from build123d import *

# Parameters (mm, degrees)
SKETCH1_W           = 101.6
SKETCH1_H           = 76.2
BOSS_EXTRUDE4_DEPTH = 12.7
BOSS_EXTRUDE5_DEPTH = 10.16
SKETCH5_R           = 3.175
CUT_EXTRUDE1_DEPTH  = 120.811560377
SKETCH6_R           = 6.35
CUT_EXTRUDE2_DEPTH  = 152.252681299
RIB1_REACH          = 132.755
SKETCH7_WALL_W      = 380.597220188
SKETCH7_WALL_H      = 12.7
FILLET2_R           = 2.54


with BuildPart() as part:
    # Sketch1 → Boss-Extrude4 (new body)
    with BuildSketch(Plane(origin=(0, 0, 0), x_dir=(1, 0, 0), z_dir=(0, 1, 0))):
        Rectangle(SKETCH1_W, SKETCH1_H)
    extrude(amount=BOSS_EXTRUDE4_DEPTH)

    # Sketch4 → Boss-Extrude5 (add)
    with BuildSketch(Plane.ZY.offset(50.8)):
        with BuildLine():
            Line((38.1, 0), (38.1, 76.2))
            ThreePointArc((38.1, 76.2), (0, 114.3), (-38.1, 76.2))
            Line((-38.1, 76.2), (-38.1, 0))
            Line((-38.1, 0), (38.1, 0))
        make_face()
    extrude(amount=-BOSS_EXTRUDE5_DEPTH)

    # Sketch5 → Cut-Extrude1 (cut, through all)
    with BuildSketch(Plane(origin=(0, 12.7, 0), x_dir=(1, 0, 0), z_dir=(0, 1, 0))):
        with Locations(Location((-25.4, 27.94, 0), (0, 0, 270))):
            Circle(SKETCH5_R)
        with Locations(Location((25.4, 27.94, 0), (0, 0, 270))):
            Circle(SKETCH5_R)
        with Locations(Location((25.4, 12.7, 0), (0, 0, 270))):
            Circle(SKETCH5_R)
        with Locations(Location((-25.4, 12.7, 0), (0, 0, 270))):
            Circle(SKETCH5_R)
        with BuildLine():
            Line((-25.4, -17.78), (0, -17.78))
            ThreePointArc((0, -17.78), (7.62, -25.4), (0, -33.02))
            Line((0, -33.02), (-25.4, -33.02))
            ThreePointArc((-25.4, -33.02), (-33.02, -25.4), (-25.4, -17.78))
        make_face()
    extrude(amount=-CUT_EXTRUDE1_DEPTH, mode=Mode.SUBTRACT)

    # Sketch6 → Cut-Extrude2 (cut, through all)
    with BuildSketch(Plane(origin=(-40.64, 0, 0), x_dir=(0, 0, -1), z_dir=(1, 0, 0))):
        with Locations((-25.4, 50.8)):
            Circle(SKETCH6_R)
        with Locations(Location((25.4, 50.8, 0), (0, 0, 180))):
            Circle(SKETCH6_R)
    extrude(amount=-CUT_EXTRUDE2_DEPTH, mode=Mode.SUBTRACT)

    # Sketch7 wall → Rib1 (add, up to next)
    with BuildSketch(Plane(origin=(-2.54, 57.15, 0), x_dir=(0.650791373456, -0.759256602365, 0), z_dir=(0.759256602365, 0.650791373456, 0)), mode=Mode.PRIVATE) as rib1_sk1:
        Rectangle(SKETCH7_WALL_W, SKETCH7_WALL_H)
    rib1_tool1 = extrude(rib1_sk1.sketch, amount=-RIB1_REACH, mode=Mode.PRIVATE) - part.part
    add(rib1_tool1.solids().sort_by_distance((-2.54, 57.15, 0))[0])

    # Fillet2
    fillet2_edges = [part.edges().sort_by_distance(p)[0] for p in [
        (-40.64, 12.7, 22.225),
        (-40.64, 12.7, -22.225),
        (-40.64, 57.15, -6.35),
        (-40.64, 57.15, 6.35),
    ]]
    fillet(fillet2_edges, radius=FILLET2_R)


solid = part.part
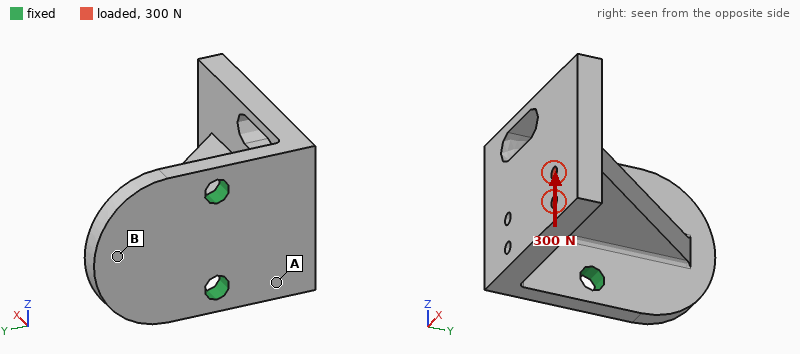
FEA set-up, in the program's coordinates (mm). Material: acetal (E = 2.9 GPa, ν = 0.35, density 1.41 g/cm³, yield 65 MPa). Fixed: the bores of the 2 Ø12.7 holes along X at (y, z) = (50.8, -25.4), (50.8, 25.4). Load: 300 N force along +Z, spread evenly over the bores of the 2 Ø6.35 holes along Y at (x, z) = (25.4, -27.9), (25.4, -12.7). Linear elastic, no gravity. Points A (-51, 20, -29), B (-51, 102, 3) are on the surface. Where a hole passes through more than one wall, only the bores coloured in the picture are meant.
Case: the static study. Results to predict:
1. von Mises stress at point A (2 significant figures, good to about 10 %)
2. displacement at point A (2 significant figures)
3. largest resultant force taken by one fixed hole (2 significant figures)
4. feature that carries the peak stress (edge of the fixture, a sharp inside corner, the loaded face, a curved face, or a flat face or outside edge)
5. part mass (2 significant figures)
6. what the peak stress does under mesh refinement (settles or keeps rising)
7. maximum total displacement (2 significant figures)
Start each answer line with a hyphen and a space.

- 4.1 MPa
- 0.15 mm
- 540 N
- edge of the fixture
- 290 g
- keeps rising
- 0.76 mm
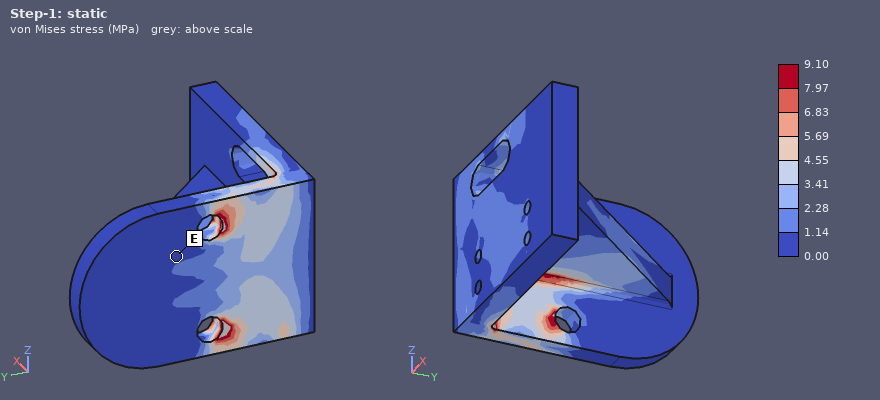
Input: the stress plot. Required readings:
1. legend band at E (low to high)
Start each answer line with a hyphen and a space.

- 0.00 to 1.14 MPa
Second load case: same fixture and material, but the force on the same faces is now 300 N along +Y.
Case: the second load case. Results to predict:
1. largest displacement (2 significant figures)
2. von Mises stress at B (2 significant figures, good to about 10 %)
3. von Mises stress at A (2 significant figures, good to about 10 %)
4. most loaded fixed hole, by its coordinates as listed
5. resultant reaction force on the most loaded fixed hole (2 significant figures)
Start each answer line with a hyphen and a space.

- 0.92 mm
- 1.4 MPa
- 1.4 MPa
- (50.8, -25.4)
- 260 N
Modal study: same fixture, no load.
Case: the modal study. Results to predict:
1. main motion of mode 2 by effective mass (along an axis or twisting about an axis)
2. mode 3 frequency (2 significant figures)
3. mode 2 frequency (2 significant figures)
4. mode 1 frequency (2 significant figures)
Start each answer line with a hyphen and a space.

- along Z
- 920 Hz
- 380 Hz
- 330 Hz
